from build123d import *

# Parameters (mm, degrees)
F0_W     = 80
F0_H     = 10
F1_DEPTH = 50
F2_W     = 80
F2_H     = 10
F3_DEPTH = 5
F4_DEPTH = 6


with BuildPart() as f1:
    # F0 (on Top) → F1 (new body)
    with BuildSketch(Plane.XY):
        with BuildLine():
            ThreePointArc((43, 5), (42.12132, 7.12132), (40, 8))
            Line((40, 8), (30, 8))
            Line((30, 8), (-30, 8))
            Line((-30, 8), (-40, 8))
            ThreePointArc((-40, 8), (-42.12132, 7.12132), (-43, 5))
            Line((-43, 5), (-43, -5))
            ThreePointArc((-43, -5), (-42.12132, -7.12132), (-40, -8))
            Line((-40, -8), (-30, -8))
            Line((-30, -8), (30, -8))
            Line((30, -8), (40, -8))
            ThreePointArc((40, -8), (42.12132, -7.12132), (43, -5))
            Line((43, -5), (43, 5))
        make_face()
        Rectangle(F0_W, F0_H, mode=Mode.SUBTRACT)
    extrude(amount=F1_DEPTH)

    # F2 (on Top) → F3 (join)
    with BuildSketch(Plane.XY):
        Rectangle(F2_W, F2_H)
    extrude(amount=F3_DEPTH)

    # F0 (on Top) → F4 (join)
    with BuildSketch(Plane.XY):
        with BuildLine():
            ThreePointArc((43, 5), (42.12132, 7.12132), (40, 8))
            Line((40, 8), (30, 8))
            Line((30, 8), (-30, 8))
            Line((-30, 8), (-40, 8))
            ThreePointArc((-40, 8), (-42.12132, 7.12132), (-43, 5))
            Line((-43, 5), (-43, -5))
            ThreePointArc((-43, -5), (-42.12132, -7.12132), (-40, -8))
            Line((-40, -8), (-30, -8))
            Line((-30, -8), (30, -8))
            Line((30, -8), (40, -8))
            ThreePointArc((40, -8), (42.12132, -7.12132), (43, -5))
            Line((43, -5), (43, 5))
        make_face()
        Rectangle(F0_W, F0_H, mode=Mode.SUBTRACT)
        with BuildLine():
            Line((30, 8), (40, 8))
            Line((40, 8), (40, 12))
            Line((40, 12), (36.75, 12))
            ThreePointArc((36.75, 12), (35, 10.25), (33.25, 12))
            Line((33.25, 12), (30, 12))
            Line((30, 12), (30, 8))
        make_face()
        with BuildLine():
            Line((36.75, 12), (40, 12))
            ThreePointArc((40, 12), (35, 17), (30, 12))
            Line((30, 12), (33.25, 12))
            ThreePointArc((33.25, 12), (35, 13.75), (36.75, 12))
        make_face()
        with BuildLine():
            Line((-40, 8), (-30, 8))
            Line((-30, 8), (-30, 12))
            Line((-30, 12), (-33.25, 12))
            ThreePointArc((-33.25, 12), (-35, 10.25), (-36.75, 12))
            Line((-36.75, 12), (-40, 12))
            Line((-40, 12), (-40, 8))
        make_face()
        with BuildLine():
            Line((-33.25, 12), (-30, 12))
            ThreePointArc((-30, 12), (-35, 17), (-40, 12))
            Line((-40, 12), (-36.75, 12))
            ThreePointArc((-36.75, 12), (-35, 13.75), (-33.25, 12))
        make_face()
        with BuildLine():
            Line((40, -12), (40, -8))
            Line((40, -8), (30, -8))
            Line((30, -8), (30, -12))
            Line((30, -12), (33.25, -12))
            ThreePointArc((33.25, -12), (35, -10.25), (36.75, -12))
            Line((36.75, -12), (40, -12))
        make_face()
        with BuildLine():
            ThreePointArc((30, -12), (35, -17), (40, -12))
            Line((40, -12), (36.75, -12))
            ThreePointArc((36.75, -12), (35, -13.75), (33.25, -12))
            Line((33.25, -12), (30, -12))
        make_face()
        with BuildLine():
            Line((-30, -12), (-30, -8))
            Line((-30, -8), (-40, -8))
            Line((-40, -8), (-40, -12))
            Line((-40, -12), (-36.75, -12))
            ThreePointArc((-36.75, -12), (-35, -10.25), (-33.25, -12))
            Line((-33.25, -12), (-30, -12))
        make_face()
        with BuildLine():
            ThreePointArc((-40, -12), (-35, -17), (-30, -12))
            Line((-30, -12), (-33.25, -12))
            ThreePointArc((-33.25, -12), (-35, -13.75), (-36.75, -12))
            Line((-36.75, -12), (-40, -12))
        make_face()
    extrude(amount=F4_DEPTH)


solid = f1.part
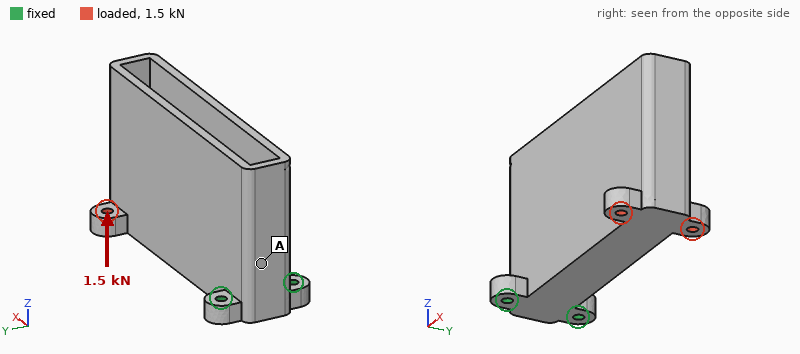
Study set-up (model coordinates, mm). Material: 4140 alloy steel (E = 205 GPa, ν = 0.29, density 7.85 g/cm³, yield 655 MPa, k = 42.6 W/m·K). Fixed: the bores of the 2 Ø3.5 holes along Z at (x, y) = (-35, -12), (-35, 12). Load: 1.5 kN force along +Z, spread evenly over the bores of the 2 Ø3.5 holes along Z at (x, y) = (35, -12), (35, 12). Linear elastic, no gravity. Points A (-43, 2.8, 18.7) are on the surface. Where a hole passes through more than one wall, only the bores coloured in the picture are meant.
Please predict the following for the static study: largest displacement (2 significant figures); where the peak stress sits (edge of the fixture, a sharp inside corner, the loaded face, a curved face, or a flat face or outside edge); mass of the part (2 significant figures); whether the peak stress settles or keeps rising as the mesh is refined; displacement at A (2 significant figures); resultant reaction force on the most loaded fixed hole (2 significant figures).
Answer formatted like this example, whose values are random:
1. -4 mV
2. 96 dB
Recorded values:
1. 0.71 mm
2. edge of the fixture
3. 270 g
4. keeps rising
5. 0.13 mm
6. 790 N
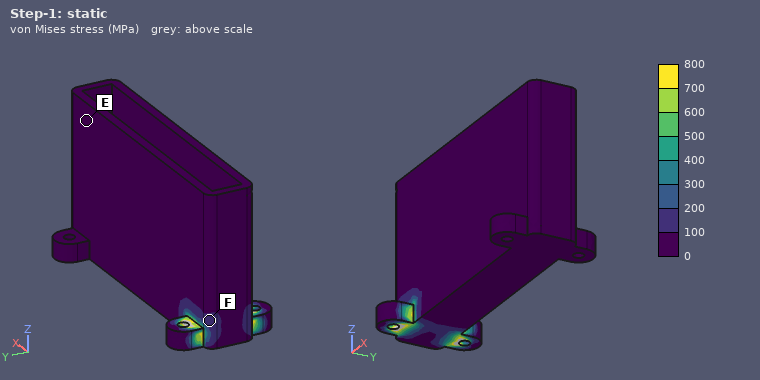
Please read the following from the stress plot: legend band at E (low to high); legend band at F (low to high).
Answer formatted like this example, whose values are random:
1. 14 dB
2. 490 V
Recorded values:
1. 0 to 100 MPa
2. 100 to 200 MPa
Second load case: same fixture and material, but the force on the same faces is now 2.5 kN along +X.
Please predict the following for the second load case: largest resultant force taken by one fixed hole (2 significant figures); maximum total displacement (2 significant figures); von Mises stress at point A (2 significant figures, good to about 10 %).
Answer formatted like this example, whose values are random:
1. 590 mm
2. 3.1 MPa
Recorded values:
1. 1.3 kN
2. 16 µm
3. 7.2 MPa
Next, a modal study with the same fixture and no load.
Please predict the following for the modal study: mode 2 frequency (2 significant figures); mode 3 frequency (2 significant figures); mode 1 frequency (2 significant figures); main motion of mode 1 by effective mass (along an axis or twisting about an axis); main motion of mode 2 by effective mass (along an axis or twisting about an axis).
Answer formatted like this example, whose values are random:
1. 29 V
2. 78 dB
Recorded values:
1. 930 Hz
2. 2400 Hz
3. 710 Hz
4. along Z
5. along Y
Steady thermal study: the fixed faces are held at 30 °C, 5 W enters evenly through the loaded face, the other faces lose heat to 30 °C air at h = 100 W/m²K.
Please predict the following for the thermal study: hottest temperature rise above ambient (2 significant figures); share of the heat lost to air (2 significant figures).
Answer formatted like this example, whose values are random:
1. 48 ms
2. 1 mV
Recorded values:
1. 16 K
2. 96 %
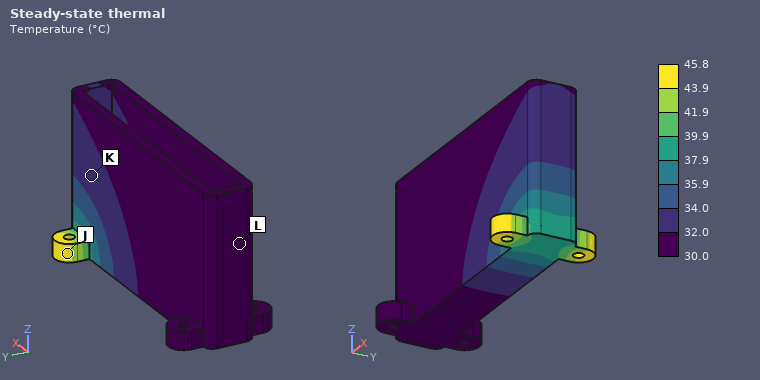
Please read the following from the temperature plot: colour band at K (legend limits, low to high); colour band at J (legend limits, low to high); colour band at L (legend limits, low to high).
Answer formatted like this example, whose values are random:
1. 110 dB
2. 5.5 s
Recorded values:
1. 32.0 to 34.0 °C
2. 43.9 to 45.8 °C
3. 30.0 to 32.0 °C
